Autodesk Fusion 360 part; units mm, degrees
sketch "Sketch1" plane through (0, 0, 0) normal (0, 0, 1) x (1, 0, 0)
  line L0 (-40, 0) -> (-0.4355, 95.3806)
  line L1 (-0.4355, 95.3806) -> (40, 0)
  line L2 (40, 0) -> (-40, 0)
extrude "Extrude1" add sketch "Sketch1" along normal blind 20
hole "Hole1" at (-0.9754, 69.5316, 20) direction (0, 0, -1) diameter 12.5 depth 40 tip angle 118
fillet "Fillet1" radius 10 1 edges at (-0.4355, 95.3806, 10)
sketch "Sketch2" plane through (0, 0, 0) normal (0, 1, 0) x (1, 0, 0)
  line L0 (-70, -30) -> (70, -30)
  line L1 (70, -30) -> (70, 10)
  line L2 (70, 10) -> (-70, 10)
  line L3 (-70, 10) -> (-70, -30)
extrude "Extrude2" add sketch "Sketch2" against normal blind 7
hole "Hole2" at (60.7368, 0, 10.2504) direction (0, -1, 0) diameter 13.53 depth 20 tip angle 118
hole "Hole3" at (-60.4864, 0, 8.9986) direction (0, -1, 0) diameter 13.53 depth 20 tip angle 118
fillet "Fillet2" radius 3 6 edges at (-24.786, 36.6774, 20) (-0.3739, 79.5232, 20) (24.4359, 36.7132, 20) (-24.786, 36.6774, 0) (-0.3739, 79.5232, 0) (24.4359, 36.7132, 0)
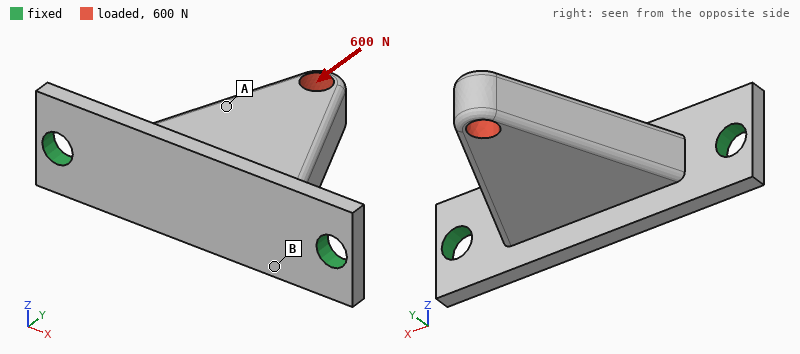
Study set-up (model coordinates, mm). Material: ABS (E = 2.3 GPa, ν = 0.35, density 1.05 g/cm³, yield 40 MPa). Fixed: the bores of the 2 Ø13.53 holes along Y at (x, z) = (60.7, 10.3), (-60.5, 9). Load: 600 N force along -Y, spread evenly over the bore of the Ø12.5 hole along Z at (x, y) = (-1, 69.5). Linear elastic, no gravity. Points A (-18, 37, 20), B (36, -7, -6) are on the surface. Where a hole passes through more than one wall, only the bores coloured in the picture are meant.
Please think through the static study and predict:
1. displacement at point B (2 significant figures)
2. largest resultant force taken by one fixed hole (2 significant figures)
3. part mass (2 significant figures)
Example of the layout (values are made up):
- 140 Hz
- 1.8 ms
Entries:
- 0.14 mm
- 360 N
- 110 g
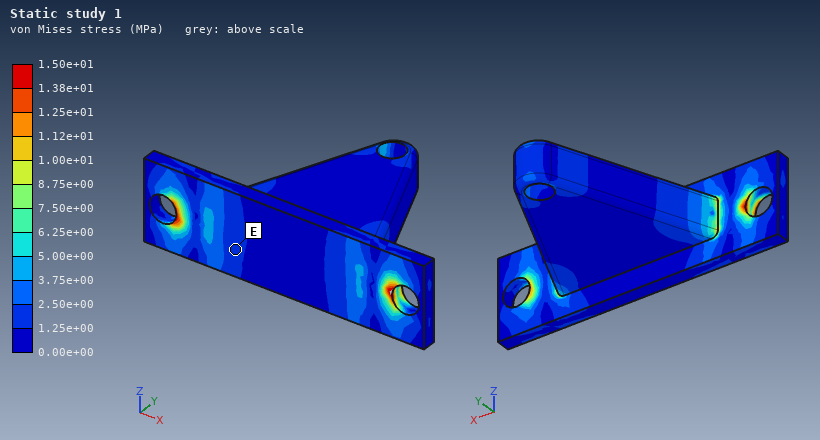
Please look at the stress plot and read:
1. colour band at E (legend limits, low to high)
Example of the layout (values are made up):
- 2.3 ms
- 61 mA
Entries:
- 1.25e+00 to 2.50e+00 MPa
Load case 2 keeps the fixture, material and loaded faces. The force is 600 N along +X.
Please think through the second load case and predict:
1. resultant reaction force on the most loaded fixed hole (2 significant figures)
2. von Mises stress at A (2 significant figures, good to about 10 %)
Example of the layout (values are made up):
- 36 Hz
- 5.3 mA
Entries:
- 560 N
- 2.1 MPa
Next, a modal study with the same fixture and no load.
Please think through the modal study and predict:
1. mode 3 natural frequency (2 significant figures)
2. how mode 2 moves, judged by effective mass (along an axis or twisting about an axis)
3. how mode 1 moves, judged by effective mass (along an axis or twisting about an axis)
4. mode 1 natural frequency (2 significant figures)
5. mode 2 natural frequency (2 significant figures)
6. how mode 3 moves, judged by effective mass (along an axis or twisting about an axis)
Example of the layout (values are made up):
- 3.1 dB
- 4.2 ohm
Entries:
- 1200 Hz
- along Y
- along Z
- 300 Hz
- 950 Hz
- along X
